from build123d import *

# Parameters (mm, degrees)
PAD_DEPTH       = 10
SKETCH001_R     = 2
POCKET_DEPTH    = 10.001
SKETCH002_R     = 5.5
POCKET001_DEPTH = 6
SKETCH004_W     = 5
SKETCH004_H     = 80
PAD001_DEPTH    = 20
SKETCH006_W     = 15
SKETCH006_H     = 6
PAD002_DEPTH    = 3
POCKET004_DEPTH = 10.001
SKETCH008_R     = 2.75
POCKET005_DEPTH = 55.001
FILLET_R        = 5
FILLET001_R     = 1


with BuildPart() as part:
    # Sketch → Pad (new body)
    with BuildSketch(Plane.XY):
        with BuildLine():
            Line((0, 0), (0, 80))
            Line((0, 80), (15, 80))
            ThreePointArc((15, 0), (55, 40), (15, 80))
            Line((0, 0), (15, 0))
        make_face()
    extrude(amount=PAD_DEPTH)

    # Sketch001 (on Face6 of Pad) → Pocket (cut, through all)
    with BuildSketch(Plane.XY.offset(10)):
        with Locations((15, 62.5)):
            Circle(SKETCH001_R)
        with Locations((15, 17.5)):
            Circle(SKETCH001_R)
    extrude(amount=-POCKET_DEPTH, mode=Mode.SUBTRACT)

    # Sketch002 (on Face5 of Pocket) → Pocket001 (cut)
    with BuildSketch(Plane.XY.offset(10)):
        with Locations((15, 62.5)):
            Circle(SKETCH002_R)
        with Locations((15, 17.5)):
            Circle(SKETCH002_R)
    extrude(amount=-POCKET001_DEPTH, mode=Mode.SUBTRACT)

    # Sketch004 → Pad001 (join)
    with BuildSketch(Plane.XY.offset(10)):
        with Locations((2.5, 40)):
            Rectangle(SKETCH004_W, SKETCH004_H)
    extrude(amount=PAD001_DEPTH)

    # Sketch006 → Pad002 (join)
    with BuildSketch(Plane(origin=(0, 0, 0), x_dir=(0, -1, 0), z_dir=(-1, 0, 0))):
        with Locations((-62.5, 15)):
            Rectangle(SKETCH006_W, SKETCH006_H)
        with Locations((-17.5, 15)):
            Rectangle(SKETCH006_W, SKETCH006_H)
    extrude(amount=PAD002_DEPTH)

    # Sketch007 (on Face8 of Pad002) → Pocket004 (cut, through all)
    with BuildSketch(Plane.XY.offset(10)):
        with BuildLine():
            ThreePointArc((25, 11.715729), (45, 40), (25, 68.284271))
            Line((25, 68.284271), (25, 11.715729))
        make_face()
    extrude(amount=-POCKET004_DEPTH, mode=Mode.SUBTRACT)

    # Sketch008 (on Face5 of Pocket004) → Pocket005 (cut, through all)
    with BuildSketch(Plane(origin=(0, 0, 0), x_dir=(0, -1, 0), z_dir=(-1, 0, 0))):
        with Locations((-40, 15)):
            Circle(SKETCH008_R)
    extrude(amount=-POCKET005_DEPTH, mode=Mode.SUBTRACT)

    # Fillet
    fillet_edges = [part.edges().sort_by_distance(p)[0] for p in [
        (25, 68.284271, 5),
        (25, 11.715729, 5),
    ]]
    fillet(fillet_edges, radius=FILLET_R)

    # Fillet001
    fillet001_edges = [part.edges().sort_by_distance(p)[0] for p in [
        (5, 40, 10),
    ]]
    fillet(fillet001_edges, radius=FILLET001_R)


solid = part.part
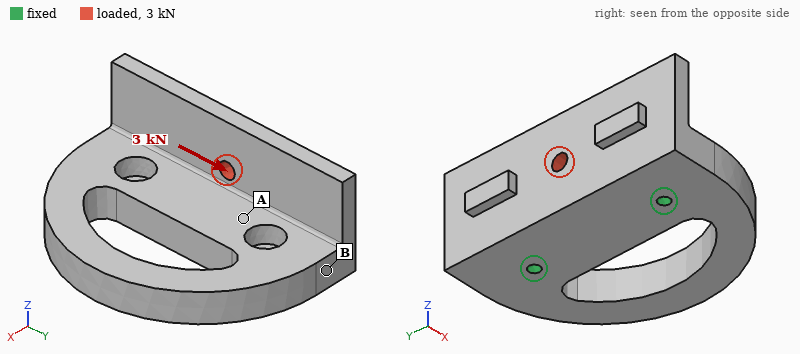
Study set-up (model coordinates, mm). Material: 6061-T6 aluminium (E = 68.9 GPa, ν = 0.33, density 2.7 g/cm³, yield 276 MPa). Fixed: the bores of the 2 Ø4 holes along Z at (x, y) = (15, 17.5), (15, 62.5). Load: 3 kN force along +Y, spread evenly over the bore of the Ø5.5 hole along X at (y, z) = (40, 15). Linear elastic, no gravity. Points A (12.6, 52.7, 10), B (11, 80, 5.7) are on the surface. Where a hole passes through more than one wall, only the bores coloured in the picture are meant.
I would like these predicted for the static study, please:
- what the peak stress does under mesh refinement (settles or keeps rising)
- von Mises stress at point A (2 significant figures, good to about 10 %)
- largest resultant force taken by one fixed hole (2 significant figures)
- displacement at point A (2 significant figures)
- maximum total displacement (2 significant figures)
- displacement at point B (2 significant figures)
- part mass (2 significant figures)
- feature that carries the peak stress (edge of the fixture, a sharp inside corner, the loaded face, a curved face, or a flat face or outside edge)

keeps rising
14 MPa
1.9 kN
4.8 µm
25 µm
12 µm
98 g
edge of the fixture
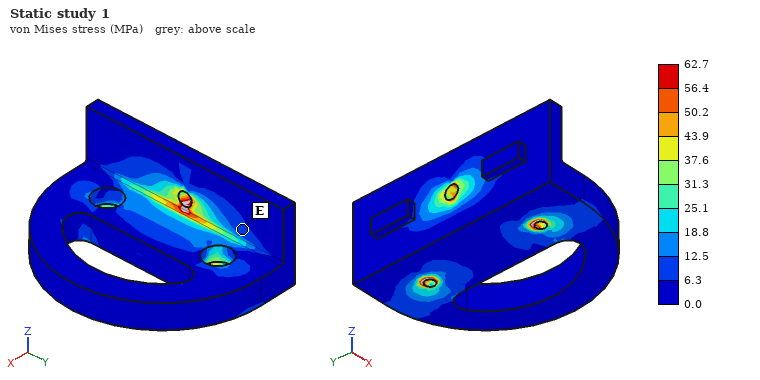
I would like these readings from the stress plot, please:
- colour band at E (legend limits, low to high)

6.3 to 12.5 MPa
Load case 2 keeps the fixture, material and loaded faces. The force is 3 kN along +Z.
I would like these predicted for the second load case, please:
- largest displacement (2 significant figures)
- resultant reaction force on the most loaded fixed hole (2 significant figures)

0.19 mm
1.6 kN
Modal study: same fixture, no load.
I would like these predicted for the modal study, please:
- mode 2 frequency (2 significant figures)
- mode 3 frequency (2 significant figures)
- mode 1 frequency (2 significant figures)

5000 Hz
5500 Hz
2100 Hz
